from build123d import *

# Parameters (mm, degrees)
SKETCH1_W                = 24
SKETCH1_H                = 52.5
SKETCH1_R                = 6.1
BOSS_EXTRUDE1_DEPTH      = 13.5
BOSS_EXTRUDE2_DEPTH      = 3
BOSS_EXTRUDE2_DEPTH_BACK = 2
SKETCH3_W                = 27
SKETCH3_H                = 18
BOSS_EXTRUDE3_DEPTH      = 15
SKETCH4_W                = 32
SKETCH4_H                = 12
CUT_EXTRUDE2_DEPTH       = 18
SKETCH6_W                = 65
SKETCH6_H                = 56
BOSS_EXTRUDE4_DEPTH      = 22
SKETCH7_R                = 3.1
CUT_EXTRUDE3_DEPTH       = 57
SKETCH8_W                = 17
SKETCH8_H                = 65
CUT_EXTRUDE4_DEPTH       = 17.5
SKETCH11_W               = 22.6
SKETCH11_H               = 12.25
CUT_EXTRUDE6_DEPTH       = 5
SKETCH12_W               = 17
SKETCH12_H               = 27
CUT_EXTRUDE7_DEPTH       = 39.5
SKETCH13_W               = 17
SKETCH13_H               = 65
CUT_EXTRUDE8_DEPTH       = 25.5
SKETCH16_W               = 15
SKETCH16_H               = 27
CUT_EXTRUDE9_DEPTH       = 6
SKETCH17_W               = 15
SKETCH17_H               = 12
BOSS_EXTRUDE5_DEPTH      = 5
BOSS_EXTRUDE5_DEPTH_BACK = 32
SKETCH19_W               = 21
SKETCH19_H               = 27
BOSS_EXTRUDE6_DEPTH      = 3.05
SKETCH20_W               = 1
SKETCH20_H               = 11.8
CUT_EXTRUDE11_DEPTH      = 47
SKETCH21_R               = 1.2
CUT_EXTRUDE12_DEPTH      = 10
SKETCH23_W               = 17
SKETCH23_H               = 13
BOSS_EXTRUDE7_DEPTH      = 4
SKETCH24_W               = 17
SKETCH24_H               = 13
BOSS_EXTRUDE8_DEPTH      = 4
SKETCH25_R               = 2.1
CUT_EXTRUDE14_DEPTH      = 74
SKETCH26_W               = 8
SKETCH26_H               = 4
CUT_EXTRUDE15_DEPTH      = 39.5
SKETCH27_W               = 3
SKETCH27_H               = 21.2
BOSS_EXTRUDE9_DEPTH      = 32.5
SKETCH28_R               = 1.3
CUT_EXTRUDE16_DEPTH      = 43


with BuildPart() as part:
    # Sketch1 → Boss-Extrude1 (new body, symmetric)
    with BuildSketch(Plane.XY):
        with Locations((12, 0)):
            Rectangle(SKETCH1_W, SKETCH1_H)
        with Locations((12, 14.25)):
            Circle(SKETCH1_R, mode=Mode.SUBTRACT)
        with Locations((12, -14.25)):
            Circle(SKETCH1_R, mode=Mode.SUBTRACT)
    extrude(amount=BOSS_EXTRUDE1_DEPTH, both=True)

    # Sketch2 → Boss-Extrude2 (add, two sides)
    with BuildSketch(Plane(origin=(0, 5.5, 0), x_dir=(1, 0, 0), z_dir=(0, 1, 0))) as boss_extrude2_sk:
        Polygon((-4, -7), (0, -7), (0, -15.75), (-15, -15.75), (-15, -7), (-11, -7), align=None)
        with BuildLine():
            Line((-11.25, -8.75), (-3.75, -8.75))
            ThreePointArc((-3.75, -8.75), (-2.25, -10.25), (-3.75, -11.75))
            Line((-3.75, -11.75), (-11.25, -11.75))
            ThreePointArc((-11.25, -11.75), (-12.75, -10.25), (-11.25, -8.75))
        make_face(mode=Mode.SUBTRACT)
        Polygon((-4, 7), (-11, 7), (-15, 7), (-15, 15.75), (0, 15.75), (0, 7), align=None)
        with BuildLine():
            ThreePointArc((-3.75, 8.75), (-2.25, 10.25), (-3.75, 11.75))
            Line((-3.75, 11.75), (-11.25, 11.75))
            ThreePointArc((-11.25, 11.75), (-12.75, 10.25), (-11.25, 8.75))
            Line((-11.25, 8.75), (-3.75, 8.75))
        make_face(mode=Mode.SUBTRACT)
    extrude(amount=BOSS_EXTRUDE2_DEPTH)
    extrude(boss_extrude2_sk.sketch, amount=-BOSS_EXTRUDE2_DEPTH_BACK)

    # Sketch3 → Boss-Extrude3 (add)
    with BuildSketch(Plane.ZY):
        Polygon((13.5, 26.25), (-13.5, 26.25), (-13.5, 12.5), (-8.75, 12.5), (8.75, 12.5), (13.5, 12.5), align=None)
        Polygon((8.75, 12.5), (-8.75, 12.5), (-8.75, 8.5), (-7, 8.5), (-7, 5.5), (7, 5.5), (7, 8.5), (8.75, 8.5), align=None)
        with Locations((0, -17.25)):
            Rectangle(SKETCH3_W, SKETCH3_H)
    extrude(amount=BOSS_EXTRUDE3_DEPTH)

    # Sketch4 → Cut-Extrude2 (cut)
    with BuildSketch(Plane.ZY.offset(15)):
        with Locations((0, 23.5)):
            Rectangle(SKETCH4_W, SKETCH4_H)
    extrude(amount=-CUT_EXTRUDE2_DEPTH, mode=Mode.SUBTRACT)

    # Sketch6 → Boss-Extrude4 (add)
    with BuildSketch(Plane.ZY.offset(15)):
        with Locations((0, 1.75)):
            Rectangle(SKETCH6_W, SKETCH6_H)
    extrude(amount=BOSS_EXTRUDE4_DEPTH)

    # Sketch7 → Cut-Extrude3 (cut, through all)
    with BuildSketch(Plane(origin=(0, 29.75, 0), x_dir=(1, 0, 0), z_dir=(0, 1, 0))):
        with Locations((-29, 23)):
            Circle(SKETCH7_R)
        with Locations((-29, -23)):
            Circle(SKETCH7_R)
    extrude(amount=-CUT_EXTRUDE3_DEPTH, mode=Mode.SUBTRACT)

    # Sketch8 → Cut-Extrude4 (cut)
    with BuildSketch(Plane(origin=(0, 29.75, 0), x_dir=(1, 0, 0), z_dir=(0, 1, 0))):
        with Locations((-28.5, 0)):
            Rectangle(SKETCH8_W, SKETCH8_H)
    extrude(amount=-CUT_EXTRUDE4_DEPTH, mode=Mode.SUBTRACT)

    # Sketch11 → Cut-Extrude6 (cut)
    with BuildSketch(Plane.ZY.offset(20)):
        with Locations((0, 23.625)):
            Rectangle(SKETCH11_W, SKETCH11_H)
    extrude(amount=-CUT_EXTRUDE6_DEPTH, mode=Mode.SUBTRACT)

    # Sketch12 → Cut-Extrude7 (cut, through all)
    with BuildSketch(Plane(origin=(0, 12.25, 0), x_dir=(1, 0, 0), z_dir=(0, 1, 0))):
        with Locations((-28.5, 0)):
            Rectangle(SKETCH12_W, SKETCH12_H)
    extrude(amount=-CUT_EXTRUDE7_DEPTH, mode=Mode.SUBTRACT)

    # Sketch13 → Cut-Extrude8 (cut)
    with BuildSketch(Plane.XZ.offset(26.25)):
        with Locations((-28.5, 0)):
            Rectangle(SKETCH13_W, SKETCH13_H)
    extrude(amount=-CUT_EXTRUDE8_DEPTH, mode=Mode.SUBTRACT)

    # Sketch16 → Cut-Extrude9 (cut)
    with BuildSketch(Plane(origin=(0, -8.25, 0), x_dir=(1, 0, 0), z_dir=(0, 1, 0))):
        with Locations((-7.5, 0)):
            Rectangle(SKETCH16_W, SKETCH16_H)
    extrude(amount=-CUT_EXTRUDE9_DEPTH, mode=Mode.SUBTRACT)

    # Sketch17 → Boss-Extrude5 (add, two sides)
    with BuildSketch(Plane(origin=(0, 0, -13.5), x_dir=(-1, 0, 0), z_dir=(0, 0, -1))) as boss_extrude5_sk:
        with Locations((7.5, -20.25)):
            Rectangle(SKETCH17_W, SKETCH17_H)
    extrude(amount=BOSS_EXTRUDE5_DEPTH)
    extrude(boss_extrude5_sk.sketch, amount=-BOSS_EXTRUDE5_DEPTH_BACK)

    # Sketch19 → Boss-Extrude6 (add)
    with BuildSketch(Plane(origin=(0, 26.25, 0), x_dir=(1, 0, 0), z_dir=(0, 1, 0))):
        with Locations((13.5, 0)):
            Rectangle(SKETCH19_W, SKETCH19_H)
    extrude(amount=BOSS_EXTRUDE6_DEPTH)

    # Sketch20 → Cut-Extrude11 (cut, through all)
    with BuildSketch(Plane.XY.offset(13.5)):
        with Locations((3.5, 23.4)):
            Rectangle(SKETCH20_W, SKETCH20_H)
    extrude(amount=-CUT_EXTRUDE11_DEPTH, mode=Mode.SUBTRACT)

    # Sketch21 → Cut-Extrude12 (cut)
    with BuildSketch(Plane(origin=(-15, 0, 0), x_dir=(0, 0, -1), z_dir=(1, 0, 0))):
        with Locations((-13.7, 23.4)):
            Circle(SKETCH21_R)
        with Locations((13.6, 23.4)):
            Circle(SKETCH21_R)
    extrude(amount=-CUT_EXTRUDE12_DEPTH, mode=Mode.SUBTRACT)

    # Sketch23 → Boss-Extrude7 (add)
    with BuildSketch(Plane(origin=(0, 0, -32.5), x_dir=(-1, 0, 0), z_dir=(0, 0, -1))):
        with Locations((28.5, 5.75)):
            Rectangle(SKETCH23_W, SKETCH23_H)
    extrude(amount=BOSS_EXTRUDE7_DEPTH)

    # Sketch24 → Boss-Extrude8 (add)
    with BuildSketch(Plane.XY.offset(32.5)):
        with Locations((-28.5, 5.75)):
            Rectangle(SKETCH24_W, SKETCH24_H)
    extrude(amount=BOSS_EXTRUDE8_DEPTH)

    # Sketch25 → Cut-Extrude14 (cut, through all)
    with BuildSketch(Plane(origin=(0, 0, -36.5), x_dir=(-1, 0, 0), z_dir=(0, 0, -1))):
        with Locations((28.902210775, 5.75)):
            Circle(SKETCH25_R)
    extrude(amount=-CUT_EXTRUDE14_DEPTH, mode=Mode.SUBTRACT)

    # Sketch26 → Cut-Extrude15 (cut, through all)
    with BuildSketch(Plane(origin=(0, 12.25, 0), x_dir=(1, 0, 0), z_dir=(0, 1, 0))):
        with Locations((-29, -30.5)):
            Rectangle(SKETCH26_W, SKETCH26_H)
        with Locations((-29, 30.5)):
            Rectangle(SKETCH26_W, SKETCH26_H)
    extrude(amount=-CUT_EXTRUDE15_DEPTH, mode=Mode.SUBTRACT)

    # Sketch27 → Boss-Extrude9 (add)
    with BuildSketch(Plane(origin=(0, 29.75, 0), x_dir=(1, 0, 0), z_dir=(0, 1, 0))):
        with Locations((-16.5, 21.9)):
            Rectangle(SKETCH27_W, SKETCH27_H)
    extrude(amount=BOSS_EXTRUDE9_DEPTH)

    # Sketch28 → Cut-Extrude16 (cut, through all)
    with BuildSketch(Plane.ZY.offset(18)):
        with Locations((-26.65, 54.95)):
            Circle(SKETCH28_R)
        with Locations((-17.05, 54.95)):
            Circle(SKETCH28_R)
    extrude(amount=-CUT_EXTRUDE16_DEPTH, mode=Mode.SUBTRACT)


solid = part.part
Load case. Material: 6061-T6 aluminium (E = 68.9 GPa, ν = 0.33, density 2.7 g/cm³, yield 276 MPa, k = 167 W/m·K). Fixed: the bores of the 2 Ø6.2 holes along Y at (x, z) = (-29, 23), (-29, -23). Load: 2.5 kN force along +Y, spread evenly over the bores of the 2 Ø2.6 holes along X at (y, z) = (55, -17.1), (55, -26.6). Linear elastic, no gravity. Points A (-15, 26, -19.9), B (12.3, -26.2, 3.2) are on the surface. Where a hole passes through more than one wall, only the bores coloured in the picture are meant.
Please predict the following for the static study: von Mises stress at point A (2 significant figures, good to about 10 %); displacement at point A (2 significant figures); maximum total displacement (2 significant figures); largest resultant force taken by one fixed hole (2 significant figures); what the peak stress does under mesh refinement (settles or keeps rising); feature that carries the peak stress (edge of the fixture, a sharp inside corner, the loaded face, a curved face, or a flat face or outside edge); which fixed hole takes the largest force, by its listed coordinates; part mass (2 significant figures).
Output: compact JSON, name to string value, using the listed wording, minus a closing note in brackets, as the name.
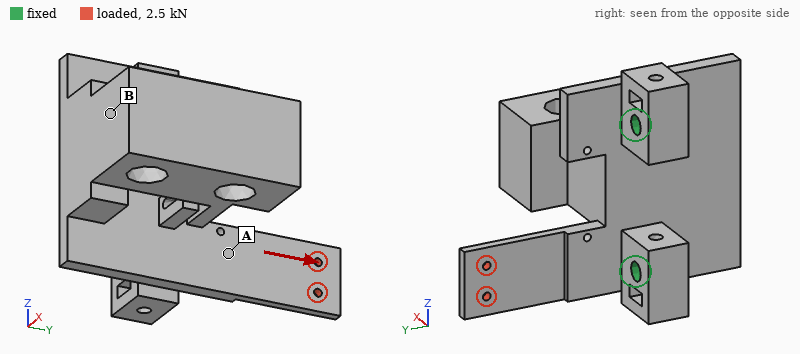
{"von Mises stress at point A": "53 MPa", "displacement at point A": "0.039 mm", "maximum total displacement": "0.18 mm", "largest resultant force taken by one fixed hole": "2.3 kN", "what the peak stress does under mesh refinement": "keeps rising", "feature that carries the peak stress": "a sharp inside corner", "which fixed hole takes the largest force, by its listed coordinates": "(-29, -23)", "part mass": "180 g"}
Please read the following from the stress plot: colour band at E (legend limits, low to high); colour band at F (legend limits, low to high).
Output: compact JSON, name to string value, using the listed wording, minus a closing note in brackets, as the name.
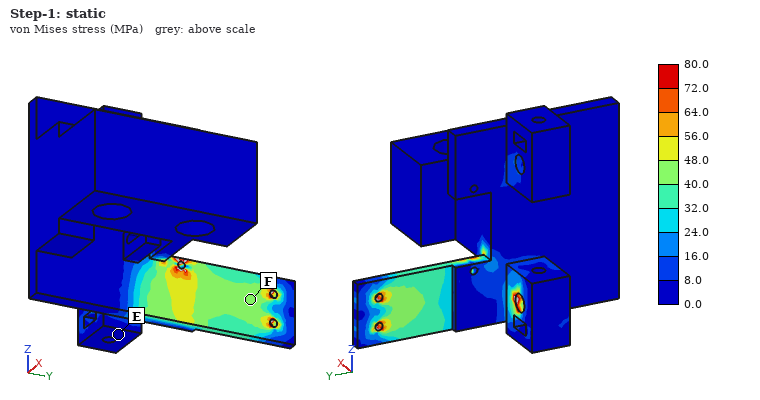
{"colour band at E": "0.0 to 8.0 MPa", "colour band at F": "40.0 to 48.0 MPa"}
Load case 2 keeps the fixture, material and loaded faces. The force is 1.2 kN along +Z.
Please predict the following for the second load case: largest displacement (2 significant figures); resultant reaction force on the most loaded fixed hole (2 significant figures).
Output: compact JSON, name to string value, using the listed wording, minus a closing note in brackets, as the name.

{"largest displacement": "0.29 mm", "resultant reaction force on the most loaded fixed hole": "1.2 kN"}
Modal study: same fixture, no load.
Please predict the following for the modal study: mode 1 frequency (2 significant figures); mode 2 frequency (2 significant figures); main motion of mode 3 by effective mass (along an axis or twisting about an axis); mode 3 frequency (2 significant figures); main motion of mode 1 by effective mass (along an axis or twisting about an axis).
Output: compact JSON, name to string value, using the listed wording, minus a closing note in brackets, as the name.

{"mode 1 frequency": "1500 Hz", "mode 2 frequency": "1700 Hz", "main motion of mode 3 by effective mass": "along Z", "mode 3 frequency": "4100 Hz", "main motion of mode 1 by effective mass": "along Y"}
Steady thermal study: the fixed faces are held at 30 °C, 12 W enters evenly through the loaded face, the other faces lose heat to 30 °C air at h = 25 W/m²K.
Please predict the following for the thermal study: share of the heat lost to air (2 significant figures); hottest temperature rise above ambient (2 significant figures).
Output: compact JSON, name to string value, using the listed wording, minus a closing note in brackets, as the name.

{"share of the heat lost to air": "17 %", "hottest temperature rise above ambient": "43 K"}
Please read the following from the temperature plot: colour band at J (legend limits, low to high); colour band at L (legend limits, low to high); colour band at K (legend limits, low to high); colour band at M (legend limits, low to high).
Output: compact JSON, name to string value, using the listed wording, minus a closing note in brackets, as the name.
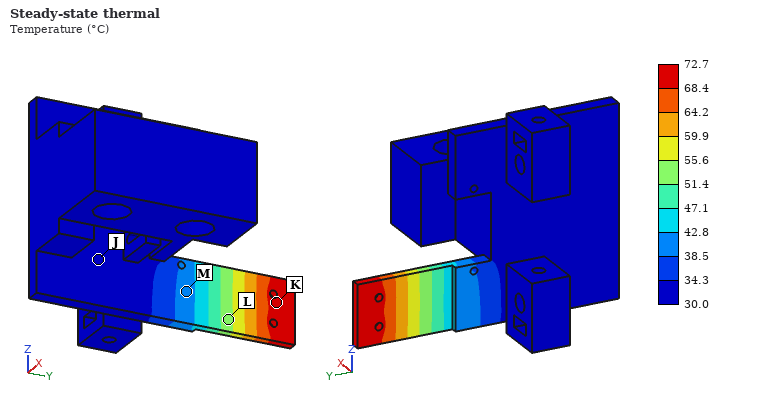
{"colour band at J": "30.0 to 34.3 °C", "colour band at L": "51.4 to 55.6 °C", "colour band at K": "68.4 to 72.7 °C", "colour band at M": "38.5 to 42.8 °C"}
